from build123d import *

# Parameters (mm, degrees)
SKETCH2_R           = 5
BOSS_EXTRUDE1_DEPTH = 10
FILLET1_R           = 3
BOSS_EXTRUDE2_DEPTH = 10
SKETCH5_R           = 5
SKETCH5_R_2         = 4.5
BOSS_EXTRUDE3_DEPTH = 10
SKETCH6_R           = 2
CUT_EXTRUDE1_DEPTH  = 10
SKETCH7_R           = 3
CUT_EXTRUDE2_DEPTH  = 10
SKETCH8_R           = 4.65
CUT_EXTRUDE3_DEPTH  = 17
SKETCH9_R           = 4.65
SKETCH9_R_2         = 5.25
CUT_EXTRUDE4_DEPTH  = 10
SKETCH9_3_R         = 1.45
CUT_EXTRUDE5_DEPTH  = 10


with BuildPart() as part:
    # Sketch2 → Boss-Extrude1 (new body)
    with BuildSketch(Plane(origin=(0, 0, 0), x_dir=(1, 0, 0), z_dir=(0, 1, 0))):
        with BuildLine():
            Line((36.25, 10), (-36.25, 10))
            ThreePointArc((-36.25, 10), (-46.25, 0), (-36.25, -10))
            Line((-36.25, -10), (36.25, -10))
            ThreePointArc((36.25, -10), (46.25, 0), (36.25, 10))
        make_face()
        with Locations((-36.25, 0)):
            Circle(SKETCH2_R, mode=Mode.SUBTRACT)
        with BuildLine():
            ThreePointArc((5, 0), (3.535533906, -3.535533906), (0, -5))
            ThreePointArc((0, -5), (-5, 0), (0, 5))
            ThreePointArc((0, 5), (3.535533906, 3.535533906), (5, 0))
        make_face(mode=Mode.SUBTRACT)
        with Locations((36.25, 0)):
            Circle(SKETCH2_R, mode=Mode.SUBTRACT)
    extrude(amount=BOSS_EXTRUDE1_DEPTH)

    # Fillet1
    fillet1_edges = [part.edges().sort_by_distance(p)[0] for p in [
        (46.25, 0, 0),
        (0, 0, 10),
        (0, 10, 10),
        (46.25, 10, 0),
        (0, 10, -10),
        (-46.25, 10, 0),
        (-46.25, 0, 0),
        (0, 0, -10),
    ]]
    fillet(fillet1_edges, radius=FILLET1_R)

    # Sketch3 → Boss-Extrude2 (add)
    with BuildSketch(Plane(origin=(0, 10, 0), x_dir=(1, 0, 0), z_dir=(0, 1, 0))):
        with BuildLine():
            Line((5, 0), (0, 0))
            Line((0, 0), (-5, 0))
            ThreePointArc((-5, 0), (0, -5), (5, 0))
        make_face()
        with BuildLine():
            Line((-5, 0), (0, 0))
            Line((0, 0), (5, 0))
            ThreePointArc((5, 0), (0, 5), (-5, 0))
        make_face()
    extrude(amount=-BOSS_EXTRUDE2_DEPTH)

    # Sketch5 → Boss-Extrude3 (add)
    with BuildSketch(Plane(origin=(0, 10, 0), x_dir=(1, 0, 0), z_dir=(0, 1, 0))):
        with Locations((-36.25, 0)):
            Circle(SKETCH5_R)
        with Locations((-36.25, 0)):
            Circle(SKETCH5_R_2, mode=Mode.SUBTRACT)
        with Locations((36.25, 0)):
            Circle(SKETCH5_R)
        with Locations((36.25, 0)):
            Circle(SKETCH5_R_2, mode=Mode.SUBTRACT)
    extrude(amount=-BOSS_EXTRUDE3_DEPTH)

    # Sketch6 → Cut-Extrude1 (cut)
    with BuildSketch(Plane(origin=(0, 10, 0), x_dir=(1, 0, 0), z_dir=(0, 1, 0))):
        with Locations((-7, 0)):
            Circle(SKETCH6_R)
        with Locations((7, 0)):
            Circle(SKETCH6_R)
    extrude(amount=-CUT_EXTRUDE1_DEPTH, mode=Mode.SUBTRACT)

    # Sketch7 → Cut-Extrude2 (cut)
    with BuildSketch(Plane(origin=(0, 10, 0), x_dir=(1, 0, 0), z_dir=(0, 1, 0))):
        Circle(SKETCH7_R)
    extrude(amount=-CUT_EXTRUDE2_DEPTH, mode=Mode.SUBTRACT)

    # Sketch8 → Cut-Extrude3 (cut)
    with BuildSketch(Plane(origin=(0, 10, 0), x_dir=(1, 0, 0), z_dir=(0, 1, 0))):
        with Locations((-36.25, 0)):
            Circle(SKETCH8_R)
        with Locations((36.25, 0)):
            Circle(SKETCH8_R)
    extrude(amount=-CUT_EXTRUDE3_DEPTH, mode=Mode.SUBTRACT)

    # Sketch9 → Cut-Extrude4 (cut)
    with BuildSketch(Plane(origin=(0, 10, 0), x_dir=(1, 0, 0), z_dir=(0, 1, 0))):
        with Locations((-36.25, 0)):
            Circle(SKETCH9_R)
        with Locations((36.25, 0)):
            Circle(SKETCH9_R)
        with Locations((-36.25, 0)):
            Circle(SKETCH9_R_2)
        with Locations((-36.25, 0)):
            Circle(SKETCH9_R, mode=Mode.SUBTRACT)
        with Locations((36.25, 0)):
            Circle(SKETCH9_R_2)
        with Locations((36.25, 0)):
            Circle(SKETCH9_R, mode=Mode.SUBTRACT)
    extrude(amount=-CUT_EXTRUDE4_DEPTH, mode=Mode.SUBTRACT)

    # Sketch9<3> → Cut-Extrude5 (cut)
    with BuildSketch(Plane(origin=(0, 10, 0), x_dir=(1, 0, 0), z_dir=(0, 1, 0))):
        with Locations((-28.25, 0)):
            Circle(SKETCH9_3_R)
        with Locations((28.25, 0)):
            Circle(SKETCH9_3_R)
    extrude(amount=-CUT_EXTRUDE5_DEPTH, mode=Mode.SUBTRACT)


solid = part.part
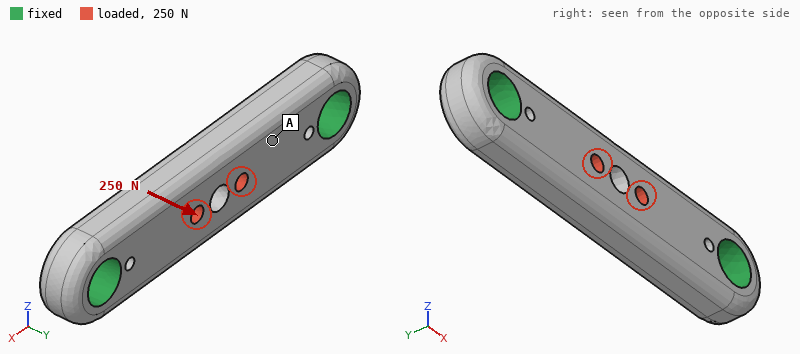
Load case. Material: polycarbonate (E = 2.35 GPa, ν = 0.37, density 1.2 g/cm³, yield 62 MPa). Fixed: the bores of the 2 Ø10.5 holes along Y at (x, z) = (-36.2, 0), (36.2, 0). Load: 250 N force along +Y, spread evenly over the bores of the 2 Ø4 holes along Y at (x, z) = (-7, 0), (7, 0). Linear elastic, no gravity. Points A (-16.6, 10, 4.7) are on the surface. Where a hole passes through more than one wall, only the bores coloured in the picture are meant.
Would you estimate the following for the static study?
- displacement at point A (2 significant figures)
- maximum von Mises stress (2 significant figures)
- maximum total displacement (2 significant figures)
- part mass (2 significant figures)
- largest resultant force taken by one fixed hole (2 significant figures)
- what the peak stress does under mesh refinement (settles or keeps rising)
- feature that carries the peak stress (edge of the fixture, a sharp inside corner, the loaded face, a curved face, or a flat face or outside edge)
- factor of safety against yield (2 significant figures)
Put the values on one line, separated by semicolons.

0.073 mm; 13 MPa; 0.13 mm; 17 g; 130 N; settles; a curved face; 4.8
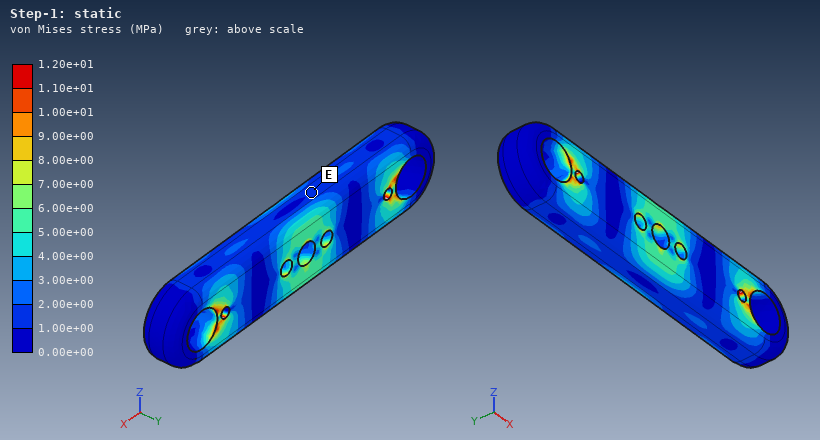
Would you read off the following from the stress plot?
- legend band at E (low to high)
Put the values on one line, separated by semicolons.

1.00e+00 to 2.00e+00 MPa
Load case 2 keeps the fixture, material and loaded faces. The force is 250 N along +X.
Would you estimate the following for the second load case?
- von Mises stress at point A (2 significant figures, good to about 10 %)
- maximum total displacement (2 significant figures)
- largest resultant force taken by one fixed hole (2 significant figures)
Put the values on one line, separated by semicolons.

0.70 MPa; 11 µm; 130 N
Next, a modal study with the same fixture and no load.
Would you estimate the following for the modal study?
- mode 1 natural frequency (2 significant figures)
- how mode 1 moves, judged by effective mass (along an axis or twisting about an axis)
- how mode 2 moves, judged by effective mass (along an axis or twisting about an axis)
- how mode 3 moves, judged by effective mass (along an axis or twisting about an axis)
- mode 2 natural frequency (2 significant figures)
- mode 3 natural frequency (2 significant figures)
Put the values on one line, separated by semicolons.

2800 Hz; along Y; along Z; twisting about X; 4000 Hz; 5100 Hz
